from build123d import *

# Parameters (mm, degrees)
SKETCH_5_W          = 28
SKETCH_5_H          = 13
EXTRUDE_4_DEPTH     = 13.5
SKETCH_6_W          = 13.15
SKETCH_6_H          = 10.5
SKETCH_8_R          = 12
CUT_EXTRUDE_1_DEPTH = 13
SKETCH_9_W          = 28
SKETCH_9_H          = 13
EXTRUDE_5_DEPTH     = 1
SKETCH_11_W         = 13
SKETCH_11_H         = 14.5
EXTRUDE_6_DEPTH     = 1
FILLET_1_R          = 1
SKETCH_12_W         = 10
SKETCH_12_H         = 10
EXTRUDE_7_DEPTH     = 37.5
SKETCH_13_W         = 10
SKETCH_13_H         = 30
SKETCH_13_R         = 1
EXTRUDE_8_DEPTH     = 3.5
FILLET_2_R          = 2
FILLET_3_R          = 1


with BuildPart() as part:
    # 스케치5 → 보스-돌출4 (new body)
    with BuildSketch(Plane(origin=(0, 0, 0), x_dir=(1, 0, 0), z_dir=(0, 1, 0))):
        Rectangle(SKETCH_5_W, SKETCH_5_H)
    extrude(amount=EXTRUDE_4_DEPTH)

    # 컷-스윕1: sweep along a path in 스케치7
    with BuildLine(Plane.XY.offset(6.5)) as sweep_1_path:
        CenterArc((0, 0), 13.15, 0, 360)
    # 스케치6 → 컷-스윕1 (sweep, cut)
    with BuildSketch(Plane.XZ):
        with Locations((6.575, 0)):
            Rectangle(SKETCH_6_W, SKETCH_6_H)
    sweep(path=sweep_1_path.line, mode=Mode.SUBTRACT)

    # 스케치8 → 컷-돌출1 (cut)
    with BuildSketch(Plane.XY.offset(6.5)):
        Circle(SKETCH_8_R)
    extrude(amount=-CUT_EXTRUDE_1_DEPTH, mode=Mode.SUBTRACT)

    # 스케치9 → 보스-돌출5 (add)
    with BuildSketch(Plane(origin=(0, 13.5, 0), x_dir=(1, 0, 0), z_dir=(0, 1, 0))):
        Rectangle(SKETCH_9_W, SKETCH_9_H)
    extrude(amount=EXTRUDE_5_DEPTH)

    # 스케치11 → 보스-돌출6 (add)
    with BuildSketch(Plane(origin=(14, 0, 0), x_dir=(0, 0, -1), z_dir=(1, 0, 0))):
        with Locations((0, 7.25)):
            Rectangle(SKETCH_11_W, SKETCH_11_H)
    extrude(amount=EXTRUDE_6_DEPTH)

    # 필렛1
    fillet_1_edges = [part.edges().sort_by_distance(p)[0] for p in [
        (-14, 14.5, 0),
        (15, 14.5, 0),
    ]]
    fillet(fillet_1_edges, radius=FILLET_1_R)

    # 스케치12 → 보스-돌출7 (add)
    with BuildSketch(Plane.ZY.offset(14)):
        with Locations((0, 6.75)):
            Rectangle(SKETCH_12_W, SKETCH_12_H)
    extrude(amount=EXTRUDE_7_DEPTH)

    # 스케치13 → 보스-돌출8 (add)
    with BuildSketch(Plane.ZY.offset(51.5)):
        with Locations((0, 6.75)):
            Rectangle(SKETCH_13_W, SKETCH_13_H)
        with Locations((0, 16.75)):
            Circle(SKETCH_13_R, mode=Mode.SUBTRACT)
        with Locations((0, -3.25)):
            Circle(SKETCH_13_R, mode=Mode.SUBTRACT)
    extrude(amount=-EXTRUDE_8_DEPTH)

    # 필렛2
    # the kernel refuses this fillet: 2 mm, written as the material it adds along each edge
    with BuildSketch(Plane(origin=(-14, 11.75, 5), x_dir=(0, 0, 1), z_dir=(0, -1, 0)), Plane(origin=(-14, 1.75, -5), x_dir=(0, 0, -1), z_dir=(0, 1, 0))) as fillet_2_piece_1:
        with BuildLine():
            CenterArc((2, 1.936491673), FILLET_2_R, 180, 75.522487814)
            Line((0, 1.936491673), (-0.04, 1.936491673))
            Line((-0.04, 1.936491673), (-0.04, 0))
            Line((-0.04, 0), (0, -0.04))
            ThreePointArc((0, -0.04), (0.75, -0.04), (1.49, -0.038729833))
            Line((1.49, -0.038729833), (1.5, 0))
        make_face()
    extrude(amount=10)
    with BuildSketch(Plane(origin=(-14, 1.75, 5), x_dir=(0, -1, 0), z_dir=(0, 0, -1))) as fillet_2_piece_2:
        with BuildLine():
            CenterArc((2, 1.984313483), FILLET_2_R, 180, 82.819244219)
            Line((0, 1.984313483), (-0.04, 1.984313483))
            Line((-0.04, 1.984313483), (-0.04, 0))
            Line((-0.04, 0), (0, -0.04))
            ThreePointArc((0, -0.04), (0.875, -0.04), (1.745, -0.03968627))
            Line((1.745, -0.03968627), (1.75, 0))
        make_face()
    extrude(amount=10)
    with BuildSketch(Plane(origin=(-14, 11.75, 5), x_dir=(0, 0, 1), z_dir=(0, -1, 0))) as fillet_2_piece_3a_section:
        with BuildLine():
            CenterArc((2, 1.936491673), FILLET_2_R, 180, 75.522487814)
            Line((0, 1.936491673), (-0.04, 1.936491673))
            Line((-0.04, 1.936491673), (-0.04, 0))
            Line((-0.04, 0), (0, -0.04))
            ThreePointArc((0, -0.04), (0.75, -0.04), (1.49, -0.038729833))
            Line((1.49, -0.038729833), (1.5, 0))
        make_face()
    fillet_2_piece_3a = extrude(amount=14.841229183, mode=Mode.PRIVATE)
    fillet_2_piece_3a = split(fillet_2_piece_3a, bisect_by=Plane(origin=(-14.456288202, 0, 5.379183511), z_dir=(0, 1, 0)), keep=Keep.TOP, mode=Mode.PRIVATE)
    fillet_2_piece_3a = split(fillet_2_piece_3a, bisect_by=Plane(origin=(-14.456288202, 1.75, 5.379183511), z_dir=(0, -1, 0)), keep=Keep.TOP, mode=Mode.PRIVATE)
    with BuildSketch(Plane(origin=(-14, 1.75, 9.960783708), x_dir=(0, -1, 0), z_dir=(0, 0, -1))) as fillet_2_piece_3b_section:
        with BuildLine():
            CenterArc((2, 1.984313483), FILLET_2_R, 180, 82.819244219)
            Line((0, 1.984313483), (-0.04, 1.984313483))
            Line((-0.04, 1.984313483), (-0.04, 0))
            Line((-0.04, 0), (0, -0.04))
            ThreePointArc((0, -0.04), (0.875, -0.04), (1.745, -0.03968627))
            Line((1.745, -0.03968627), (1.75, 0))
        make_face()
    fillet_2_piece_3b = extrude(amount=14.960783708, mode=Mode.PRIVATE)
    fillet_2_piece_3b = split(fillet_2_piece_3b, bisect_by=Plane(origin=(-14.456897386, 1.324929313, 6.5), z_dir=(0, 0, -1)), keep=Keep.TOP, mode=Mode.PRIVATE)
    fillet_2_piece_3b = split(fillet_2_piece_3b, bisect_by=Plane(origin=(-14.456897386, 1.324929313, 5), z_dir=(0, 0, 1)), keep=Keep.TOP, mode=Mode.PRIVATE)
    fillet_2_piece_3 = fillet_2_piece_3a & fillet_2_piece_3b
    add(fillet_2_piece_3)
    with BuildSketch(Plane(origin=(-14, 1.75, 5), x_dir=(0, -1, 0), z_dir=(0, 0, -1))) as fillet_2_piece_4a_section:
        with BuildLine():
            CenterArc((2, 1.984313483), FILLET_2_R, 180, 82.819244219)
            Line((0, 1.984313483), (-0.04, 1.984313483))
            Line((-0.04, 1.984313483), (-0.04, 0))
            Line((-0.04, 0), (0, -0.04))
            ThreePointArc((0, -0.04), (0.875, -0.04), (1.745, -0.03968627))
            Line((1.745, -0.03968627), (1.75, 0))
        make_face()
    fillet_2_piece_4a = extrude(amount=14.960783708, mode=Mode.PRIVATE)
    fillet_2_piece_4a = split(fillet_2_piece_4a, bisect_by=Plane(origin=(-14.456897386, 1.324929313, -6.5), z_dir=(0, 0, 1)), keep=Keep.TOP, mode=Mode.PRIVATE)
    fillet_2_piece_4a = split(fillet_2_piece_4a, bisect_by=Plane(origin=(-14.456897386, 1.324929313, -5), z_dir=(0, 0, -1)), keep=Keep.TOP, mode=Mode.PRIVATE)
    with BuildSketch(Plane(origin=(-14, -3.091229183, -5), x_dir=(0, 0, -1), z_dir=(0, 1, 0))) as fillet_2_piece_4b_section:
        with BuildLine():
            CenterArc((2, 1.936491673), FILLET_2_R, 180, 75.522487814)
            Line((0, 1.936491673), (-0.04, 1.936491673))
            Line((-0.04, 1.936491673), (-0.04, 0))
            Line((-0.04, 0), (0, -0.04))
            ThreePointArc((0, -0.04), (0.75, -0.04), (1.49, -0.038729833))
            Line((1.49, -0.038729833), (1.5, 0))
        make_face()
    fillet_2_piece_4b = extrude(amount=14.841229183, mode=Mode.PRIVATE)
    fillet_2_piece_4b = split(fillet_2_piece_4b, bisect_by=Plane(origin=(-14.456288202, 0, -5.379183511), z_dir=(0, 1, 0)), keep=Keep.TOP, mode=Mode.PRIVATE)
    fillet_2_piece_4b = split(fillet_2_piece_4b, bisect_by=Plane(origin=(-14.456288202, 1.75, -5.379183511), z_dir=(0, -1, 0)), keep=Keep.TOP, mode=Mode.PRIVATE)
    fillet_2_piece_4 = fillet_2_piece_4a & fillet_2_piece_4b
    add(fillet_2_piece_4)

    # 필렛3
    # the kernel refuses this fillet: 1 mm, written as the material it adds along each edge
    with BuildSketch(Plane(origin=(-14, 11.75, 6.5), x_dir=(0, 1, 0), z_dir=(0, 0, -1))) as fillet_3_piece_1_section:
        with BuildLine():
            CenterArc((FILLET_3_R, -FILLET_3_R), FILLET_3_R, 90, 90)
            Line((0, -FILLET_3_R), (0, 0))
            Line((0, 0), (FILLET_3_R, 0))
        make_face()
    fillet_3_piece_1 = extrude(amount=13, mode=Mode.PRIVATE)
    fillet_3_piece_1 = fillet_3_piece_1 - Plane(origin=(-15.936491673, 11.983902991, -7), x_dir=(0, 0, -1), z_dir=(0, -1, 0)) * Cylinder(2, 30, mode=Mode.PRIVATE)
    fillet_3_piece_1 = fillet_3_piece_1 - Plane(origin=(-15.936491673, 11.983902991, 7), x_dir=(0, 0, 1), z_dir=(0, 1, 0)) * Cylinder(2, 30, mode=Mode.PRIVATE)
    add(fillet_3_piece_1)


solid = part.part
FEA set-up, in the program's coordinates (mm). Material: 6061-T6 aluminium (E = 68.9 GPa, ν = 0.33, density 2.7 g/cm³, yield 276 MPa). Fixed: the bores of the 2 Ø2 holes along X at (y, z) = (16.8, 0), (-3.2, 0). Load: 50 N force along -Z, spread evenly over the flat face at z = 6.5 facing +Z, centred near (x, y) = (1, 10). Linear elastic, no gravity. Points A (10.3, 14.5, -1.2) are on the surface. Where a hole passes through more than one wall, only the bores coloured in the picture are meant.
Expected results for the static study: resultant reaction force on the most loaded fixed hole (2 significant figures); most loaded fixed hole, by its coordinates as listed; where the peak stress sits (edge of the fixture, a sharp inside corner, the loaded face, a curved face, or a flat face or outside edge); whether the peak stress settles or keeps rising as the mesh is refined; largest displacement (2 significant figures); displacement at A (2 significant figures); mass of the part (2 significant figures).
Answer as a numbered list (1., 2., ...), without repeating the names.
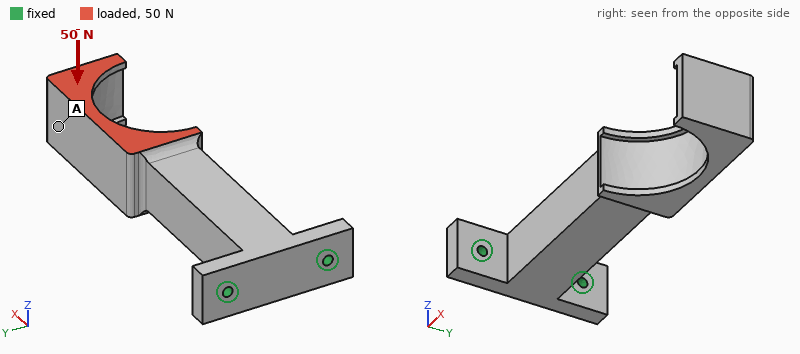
1. 33 N
2. (16.8, 0)
3. edge of the fixture
4. keeps rising
5. 0.23 mm
6. 0.19 mm
7. 18 g
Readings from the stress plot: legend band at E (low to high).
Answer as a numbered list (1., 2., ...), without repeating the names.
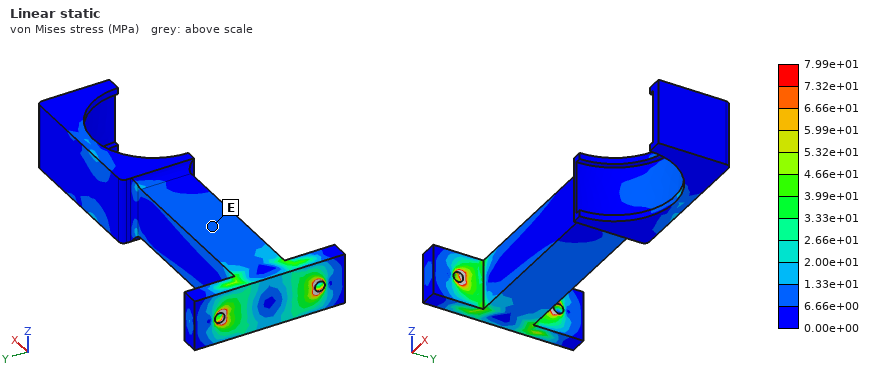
1. 6.66e+00 to 1.33e+01 MPa
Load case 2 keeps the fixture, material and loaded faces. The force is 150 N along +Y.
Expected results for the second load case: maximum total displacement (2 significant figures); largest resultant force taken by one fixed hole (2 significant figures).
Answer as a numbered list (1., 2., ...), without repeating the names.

1. 0.59 mm
2. 490 N
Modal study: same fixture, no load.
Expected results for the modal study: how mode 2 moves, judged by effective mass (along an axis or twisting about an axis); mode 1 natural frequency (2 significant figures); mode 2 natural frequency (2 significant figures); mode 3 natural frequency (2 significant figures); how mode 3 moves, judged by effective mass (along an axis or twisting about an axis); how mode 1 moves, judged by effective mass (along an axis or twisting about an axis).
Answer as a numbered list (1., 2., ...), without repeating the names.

1. along Y
2. 1000 Hz
3. 1300 Hz
4. 3200 Hz
5. along Y
6. along Z
